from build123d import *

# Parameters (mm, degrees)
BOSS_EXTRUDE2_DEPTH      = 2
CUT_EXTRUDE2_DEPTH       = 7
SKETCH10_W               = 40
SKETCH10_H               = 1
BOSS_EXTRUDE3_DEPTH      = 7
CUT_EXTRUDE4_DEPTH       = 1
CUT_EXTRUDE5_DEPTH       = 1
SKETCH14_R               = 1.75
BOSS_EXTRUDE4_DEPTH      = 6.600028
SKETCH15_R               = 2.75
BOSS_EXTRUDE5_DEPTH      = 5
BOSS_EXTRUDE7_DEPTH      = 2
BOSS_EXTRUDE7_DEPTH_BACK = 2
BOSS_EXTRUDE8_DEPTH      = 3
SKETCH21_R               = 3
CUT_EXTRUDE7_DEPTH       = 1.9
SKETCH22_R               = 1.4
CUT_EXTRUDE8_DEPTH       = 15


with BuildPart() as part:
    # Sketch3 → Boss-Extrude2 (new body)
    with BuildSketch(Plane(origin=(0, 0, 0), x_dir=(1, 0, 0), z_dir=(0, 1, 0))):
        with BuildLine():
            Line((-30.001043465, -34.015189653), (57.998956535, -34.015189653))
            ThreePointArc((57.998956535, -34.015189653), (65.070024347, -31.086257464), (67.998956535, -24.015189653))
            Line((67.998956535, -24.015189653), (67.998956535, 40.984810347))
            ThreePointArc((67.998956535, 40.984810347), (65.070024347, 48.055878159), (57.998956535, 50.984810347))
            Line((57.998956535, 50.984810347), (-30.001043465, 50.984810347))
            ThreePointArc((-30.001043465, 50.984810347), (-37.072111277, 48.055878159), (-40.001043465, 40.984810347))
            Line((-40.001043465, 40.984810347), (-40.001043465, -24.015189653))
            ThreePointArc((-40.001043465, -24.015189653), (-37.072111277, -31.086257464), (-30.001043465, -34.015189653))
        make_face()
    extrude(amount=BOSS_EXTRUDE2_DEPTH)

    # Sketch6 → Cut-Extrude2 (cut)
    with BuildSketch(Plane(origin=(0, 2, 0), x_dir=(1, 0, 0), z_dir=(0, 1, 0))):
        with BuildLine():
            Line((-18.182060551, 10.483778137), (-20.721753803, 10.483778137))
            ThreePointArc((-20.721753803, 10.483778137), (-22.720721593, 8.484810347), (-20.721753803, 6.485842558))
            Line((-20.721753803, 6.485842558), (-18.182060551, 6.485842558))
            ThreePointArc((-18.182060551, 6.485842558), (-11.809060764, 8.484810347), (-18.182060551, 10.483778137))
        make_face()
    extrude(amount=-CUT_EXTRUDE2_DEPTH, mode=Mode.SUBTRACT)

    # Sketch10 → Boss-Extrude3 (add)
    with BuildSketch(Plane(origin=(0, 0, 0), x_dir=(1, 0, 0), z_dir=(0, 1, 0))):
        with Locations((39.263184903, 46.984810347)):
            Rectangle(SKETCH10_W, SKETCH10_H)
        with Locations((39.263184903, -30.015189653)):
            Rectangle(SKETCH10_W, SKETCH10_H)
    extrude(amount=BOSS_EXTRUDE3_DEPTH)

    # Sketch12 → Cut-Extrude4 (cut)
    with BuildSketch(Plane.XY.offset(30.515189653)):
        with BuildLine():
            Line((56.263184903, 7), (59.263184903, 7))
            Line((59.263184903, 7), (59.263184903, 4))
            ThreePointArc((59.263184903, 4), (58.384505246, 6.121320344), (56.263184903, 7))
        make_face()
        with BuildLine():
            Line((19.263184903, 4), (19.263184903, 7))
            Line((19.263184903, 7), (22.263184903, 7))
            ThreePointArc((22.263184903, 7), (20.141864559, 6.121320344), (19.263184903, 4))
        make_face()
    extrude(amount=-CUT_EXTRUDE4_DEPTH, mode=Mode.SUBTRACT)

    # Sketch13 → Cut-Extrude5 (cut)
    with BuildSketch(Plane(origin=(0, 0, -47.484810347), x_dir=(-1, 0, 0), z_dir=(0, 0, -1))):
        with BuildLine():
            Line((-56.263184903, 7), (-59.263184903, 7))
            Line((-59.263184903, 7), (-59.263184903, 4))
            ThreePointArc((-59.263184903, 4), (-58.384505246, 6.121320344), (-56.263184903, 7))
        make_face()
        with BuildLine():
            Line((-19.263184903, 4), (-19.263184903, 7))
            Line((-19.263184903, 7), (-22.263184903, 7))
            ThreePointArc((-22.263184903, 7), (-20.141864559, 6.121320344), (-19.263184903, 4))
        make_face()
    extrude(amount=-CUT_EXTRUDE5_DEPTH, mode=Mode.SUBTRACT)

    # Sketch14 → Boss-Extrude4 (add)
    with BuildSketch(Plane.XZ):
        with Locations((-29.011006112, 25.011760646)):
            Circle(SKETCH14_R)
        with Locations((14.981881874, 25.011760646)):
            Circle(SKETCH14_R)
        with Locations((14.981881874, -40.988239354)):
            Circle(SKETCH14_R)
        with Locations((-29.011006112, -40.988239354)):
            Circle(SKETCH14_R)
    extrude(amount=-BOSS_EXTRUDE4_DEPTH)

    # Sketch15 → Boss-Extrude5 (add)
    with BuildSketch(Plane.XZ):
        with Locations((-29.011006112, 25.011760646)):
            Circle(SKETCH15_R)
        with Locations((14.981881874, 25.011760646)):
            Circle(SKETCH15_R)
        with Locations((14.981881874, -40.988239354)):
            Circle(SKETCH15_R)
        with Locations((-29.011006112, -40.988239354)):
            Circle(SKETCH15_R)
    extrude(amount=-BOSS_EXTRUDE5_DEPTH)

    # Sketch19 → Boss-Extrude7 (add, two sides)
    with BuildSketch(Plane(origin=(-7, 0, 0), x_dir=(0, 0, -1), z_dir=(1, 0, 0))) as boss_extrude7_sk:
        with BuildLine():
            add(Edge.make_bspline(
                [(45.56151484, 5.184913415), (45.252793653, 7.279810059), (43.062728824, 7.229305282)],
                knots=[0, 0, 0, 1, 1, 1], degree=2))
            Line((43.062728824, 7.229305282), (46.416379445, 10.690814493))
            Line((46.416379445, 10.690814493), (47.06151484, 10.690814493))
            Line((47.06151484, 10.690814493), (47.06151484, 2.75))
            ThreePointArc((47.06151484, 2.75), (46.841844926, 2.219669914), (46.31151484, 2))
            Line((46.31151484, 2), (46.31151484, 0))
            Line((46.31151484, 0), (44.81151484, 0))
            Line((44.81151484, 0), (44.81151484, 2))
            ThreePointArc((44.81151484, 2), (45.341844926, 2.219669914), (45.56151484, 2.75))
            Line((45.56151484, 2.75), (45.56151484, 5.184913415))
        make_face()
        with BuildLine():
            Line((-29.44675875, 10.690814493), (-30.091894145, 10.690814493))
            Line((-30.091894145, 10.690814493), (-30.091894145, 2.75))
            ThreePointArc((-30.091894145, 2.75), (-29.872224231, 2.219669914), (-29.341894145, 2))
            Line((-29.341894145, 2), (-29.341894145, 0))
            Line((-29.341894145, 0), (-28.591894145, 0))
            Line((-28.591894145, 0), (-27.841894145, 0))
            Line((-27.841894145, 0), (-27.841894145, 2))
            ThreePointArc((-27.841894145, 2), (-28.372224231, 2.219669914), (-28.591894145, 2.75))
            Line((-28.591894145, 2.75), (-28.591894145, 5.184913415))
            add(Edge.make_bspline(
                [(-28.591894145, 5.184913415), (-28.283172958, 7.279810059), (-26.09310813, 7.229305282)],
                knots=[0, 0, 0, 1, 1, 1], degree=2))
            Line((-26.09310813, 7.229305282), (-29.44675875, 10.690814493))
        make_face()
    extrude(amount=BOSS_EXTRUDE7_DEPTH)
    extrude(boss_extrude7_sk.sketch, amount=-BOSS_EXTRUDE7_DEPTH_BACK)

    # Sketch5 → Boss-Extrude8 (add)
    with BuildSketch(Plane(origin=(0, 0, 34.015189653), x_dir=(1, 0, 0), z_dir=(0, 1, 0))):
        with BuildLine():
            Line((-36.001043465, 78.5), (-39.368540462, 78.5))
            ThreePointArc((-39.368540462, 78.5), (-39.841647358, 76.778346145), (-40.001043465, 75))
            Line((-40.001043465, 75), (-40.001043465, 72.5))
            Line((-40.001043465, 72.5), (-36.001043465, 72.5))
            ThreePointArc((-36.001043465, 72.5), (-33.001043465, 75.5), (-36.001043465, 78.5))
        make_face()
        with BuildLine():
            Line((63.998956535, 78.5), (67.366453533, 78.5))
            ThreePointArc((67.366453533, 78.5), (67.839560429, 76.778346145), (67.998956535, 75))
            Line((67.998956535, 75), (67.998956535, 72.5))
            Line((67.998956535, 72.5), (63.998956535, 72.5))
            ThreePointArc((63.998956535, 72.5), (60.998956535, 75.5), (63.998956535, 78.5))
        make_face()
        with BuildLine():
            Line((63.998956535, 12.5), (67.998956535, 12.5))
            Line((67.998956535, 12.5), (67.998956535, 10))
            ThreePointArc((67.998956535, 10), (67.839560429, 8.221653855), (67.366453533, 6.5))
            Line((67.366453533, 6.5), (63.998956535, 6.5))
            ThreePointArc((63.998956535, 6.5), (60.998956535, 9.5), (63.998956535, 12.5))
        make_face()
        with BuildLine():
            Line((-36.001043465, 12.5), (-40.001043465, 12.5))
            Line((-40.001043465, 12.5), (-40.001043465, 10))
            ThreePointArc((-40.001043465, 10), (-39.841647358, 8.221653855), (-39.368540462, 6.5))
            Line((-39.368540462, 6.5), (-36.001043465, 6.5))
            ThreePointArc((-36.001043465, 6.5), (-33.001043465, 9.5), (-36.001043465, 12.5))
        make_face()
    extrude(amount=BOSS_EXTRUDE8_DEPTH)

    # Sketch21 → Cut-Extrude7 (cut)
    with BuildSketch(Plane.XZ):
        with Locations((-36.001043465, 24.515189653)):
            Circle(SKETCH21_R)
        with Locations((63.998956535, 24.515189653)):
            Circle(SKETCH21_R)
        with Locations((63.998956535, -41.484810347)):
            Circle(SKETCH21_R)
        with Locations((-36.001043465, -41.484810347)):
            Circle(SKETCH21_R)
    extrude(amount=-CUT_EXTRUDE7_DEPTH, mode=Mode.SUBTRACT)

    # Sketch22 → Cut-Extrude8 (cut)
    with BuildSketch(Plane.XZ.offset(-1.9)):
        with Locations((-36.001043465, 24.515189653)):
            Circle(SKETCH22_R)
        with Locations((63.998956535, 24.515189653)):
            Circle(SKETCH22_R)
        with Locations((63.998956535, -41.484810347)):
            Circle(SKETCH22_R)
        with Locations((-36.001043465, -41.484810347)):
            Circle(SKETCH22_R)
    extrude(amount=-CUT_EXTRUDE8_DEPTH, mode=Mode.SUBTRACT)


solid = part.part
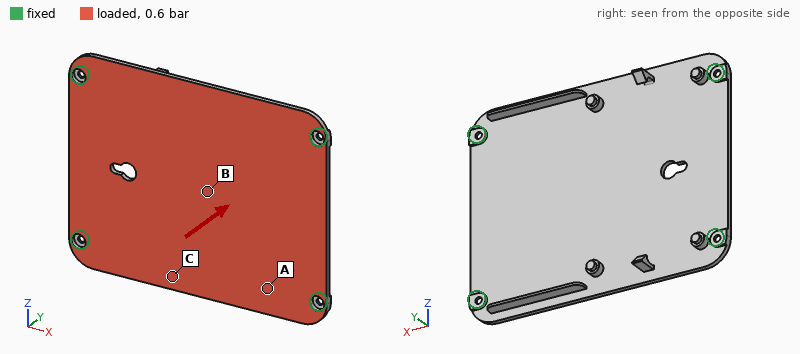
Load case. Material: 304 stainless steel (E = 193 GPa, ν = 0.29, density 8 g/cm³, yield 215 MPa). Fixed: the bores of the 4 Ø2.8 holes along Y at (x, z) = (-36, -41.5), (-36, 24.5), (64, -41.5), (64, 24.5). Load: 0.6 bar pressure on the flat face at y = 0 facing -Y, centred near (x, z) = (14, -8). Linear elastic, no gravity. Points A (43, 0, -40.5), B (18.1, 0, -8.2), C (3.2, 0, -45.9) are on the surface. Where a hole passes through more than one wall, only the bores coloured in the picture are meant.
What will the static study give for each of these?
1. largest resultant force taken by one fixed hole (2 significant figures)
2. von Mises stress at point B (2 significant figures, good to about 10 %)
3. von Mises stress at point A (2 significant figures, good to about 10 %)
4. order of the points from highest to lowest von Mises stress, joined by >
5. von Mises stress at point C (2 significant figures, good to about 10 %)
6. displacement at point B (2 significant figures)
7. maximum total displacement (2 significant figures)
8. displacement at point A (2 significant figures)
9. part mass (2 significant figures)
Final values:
520 N
43 MPa
20 MPa
C > B > A
57 MPa
0.21 mm
0.21 mm
0.089 mm
150 g
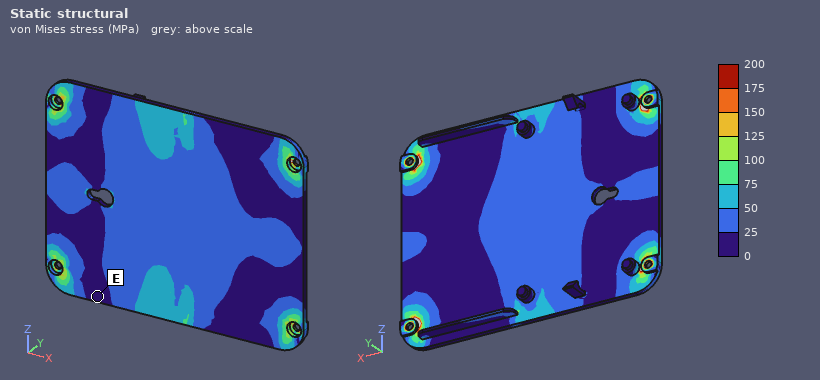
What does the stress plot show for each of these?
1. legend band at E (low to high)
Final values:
0 to 25 MPa
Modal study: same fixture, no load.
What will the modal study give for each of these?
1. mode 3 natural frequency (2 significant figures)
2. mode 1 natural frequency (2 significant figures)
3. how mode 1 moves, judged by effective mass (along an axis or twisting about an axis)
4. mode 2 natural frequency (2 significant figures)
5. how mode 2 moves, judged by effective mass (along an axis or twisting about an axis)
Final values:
1800 Hz
770 Hz
along Y
1200 Hz
twisting about X
